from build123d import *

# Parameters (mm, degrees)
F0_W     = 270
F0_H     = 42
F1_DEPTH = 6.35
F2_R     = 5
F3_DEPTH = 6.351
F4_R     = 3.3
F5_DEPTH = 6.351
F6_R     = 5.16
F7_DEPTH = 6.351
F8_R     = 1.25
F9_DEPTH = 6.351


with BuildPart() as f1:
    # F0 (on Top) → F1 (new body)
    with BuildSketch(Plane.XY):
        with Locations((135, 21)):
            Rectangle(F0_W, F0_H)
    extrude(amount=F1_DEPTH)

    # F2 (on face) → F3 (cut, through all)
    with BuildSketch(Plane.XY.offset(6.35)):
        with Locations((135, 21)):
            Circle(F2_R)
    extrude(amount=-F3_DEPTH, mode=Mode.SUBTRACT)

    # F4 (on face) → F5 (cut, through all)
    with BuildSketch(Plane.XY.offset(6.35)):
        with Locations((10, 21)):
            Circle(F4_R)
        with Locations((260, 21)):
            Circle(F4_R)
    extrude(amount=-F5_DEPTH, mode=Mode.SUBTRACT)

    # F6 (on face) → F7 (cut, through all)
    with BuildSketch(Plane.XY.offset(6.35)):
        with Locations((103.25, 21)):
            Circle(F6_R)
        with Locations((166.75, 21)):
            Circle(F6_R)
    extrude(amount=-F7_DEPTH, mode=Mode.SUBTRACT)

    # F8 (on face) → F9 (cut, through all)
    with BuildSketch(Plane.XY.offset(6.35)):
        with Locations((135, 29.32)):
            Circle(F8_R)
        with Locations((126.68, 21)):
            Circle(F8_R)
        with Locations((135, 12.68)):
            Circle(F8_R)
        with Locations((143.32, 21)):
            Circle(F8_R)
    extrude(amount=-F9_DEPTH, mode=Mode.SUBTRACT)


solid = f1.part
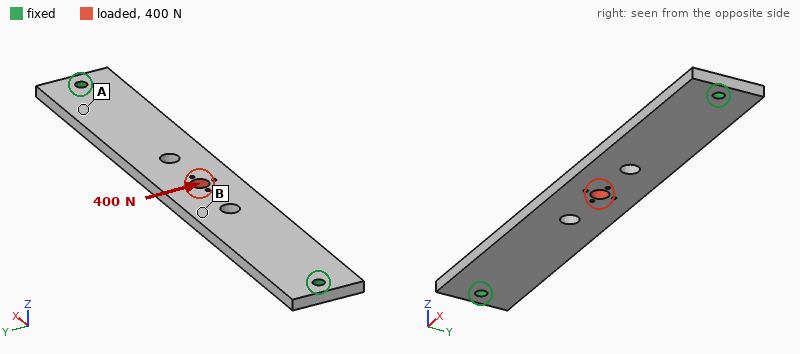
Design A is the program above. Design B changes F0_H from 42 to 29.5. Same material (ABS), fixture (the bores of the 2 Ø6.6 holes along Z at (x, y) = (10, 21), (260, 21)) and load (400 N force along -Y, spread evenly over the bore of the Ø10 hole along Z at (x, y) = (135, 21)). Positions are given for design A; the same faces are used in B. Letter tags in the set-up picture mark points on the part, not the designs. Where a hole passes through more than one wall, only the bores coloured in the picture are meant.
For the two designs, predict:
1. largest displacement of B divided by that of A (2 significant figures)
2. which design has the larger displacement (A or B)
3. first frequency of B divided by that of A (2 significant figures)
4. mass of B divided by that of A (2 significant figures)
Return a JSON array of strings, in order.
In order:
["1.9", "B", "1.0", "0.69"]
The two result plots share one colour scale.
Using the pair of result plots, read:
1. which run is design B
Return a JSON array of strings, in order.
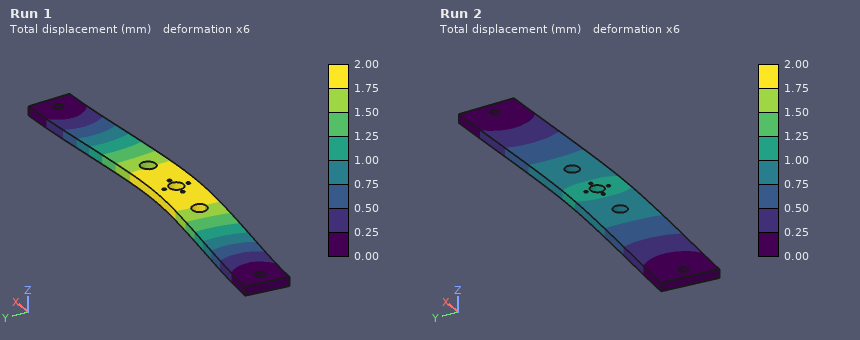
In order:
["Run 1"]
